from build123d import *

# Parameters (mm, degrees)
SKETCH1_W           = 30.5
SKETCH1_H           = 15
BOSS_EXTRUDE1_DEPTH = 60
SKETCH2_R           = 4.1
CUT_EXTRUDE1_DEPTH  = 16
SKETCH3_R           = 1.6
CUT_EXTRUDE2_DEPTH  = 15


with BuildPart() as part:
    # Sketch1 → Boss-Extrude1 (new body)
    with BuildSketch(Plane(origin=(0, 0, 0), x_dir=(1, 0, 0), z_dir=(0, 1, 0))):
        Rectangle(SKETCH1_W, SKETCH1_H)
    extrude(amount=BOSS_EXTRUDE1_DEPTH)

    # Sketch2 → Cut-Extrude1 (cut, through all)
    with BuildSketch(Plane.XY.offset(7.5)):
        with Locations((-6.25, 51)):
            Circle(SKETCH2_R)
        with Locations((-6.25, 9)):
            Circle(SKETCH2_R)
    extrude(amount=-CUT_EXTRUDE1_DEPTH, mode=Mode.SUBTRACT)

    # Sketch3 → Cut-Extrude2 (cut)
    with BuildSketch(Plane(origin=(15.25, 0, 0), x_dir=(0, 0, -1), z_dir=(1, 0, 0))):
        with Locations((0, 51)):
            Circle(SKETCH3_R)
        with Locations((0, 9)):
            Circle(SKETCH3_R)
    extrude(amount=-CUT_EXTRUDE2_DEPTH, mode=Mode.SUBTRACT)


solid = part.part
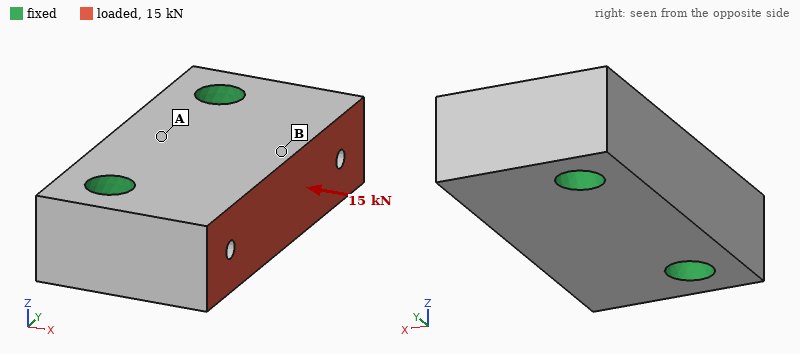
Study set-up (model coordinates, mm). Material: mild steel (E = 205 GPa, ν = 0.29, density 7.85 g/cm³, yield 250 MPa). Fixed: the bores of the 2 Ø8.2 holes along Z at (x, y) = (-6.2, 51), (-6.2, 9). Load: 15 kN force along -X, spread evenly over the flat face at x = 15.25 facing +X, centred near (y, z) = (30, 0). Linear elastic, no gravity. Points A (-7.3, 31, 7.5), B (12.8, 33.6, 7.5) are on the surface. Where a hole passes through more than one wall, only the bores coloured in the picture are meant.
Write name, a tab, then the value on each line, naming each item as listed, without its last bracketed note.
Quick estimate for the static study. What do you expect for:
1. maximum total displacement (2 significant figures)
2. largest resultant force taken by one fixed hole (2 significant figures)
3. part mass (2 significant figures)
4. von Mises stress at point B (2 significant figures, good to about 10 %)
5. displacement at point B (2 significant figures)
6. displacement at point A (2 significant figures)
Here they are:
maximum total displacement	3.1 µm
largest resultant force taken by one fixed hole	7.7 kN
part mass	200 g
von Mises stress at point B	15 MPa
displacement at point B	2.8 µm
displacement at point A	2.1 µm
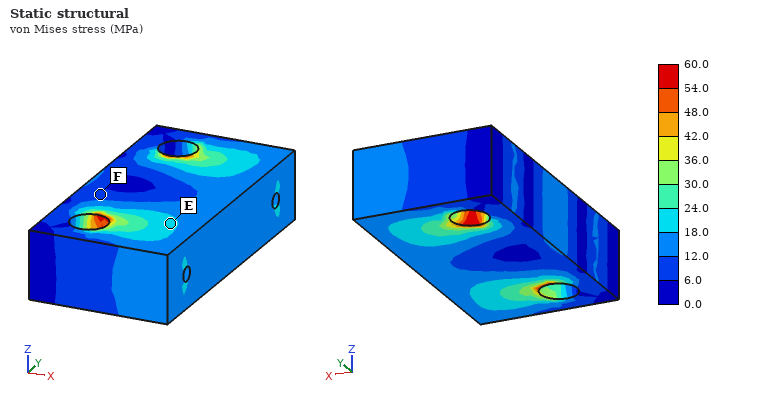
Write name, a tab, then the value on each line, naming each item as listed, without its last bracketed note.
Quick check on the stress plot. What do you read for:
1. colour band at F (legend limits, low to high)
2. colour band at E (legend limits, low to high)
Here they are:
colour band at F	6.0 to 12.0 MPa
colour band at E	18.0 to 24.0 MPa
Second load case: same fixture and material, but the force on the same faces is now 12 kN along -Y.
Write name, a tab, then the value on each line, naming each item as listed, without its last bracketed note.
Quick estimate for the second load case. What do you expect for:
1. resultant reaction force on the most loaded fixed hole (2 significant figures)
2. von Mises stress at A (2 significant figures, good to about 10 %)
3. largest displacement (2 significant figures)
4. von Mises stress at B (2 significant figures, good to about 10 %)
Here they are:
resultant reaction force on the most loaded fixed hole	7.9 kN
von Mises stress at A	10 MPa
largest displacement	7.5 µm
von Mises stress at B	28 MPa
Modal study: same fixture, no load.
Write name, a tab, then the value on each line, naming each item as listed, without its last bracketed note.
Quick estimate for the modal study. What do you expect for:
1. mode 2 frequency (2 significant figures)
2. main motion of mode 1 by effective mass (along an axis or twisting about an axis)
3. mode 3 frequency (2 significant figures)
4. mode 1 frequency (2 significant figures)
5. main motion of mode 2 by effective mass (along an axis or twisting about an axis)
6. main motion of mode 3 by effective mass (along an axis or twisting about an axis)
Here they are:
mode 2 frequency	27 kHz
main motion of mode 1 by effective mass	along Z
mode 3 frequency	30 kHz
mode 1 frequency	18 kHz
main motion of mode 2 by effective mass	twisting about X
main motion of mode 3 by effective mass	along X
